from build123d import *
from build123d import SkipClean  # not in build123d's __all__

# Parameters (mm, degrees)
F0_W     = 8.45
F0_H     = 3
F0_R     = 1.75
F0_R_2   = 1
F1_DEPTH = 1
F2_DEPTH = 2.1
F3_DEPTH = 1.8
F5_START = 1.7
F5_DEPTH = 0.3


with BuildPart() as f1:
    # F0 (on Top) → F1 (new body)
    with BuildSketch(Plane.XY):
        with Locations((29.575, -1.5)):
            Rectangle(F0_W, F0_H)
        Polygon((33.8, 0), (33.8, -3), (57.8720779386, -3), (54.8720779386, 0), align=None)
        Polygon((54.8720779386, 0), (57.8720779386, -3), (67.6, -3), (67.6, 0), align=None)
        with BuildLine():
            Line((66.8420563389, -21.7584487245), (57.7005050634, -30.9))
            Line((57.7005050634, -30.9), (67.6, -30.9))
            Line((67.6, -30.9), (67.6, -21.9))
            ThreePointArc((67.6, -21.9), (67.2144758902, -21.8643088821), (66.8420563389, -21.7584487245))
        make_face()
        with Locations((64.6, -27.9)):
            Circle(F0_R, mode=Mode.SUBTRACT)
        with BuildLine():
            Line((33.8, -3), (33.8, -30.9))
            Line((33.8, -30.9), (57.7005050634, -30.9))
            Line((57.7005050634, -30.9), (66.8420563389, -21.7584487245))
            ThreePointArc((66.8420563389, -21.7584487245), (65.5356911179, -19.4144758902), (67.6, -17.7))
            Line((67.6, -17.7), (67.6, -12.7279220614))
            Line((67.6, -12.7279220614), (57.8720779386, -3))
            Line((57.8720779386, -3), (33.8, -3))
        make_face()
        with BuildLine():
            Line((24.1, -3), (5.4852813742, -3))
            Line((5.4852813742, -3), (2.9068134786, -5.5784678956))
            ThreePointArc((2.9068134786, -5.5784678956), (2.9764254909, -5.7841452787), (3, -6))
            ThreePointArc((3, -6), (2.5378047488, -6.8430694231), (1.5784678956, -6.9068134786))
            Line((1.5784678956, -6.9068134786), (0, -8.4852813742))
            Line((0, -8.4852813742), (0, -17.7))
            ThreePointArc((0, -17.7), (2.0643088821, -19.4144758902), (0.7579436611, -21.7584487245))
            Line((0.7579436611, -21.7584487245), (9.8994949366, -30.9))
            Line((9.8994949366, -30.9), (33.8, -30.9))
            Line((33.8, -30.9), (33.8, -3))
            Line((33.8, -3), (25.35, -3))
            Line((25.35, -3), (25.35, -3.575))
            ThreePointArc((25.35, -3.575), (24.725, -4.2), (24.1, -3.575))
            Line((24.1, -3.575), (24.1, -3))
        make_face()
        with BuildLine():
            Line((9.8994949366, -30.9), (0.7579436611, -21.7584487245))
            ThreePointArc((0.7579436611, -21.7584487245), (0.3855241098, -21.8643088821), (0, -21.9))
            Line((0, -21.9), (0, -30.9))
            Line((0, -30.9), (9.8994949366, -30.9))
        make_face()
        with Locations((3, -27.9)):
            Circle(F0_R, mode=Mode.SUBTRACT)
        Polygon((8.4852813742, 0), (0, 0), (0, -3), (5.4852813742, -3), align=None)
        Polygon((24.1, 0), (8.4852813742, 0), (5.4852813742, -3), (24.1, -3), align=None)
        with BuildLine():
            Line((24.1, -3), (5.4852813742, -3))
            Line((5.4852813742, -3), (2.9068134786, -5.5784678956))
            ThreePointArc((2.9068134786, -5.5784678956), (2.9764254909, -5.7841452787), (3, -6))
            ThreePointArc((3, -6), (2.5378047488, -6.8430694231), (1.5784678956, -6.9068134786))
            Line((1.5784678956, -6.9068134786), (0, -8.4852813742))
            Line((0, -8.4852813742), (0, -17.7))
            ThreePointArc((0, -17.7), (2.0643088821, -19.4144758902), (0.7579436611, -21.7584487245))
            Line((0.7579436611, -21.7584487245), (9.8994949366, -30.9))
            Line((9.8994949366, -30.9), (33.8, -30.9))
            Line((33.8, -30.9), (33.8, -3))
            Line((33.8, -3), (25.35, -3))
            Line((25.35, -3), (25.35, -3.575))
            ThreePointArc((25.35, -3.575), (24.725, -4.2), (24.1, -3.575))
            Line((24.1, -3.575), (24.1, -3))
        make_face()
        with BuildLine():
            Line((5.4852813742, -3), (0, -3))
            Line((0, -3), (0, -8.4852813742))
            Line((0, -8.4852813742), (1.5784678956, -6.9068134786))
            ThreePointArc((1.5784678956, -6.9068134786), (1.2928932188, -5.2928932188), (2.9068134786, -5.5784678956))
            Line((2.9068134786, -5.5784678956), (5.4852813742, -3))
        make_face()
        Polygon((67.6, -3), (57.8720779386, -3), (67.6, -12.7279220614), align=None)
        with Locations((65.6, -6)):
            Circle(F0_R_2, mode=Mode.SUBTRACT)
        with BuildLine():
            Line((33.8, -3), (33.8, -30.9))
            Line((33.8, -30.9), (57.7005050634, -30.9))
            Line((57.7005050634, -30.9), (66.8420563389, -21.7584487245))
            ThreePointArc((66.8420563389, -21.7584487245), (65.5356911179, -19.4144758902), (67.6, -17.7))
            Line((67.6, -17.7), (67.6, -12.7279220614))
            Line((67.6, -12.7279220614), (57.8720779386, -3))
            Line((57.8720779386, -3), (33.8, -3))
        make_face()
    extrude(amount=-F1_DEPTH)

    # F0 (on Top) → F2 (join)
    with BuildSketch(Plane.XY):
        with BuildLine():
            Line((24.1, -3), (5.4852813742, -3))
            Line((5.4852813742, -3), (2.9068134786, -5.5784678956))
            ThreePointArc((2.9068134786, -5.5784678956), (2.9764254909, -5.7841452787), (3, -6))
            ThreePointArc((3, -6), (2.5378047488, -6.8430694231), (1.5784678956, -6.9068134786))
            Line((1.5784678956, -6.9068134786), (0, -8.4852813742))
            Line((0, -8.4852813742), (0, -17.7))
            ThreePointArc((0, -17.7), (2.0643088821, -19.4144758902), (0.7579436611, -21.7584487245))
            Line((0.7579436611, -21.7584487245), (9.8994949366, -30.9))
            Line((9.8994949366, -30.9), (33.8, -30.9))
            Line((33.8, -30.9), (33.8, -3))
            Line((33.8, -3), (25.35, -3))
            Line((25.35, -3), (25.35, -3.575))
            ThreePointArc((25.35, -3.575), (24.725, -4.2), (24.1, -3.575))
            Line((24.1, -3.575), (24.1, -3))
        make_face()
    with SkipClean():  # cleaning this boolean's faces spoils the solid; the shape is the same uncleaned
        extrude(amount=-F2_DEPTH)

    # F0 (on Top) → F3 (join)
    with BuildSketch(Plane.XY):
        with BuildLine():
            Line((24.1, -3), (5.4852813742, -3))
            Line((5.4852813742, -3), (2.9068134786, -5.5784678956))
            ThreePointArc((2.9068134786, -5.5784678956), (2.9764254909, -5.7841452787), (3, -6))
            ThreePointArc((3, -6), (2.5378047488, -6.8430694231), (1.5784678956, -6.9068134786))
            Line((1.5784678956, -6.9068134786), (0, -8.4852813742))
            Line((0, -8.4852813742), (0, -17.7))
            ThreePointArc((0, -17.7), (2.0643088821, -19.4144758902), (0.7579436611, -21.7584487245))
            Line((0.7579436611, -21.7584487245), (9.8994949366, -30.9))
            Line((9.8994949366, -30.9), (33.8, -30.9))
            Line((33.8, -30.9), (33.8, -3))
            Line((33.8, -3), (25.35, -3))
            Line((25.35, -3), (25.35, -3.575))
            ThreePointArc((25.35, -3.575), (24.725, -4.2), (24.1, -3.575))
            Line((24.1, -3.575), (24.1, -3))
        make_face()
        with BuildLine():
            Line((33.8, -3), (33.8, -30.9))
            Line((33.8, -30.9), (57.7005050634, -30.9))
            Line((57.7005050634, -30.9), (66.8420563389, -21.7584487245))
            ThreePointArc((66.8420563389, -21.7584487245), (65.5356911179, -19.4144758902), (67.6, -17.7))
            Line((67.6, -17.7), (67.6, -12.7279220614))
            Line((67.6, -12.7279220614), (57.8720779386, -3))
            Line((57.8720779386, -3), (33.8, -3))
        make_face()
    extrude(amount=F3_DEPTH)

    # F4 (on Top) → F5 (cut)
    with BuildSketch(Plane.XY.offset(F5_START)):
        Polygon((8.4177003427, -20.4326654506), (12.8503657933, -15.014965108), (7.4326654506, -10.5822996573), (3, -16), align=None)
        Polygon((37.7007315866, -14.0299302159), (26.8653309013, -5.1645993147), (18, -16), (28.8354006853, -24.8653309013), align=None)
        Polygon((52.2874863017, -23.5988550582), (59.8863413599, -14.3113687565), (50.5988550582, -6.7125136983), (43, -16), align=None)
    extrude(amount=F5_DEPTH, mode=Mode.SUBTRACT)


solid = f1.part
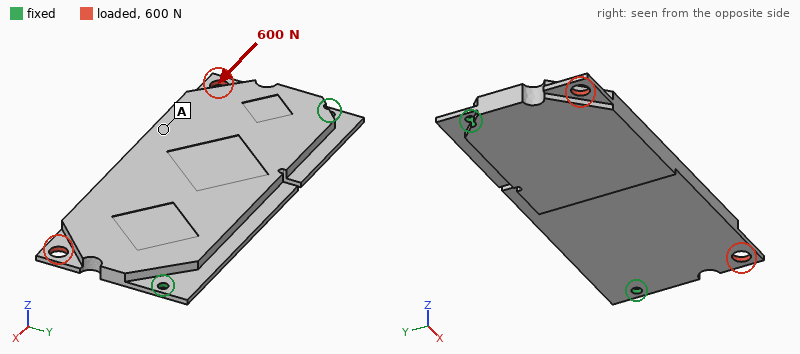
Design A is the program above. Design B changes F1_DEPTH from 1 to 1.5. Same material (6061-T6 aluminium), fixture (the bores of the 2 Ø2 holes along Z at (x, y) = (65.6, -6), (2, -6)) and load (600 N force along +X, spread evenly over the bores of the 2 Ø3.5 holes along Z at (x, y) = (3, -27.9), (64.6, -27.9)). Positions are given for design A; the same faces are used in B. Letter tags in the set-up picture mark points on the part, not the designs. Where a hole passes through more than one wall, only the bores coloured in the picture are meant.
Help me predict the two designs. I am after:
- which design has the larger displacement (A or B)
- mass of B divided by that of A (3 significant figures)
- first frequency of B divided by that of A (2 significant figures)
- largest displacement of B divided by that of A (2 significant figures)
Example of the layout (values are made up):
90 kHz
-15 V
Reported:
A
1.10
1.1
0.67
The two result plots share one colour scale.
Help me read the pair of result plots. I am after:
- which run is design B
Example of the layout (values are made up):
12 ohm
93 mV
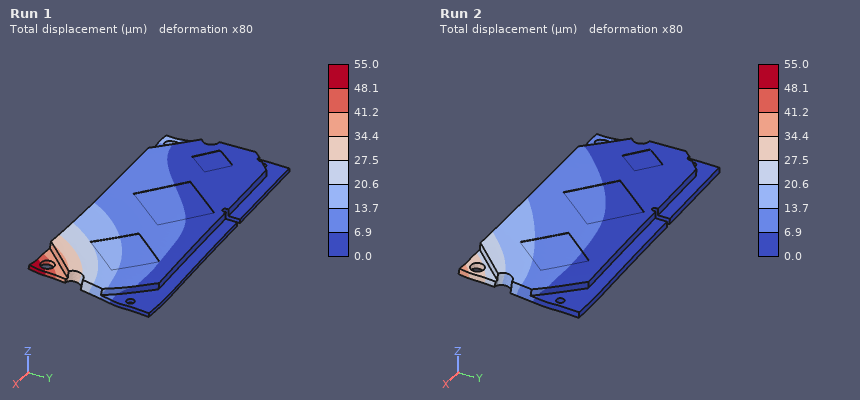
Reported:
Run 2
